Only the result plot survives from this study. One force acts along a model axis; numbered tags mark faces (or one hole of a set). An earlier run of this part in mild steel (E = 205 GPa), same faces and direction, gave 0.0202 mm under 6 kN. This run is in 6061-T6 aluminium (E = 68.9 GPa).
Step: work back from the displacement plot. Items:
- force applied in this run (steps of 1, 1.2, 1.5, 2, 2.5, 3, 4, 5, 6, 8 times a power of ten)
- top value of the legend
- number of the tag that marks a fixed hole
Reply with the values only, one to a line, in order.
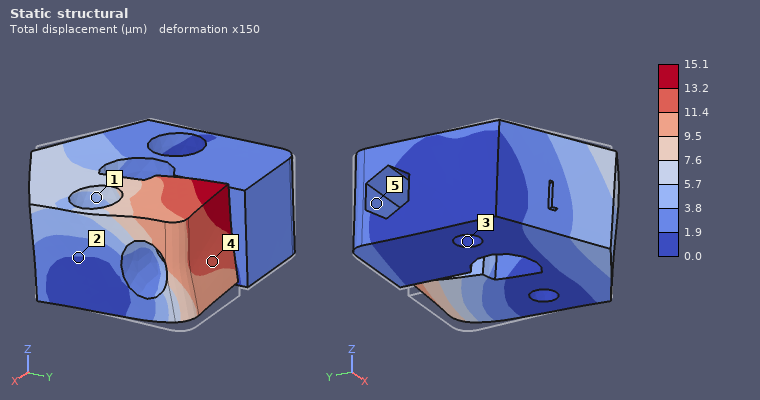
1.5 kN
15.1 µm
3
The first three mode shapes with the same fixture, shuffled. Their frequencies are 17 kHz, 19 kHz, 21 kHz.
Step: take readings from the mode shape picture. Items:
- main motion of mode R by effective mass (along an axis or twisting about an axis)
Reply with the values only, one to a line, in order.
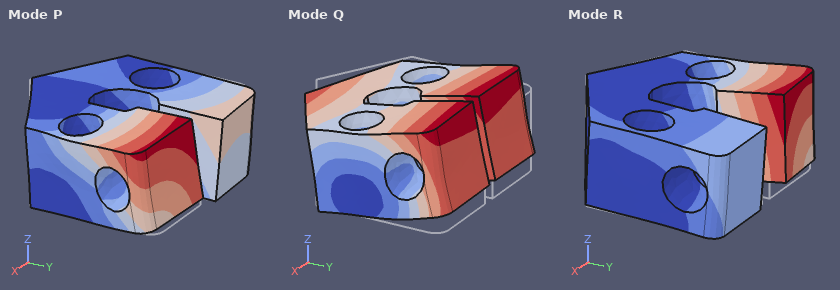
along X
